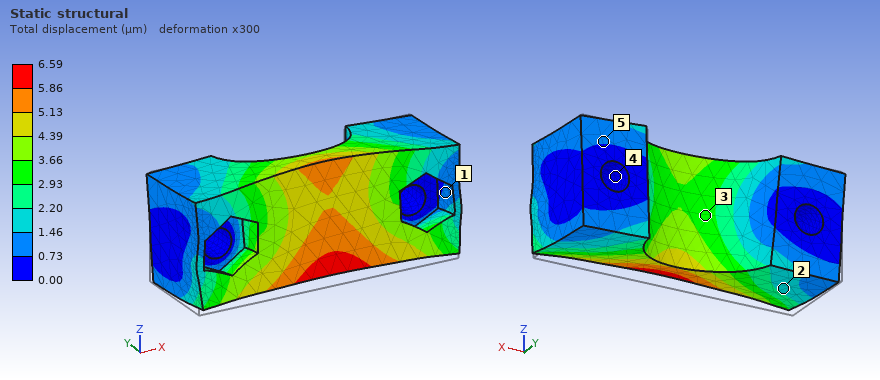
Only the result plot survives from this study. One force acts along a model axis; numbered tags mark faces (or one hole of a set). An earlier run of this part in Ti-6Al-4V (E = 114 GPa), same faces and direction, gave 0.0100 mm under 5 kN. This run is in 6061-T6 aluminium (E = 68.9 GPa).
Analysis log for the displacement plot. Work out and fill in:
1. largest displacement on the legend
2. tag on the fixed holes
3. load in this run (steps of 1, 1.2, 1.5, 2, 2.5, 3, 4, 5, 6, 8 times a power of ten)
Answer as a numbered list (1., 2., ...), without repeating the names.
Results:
1. 6.59 µm
2. 4
3. 2 kN
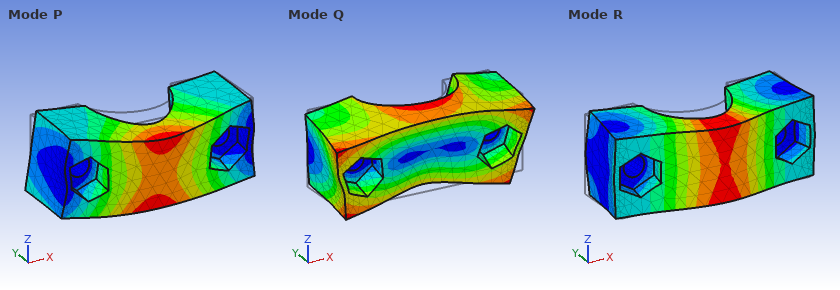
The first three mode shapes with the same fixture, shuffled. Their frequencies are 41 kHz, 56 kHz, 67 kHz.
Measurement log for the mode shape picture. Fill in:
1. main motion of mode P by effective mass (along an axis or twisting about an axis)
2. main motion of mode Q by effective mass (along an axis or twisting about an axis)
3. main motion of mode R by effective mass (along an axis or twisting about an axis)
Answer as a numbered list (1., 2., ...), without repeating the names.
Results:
1. along Z
2. twisting about X
3. along Y
